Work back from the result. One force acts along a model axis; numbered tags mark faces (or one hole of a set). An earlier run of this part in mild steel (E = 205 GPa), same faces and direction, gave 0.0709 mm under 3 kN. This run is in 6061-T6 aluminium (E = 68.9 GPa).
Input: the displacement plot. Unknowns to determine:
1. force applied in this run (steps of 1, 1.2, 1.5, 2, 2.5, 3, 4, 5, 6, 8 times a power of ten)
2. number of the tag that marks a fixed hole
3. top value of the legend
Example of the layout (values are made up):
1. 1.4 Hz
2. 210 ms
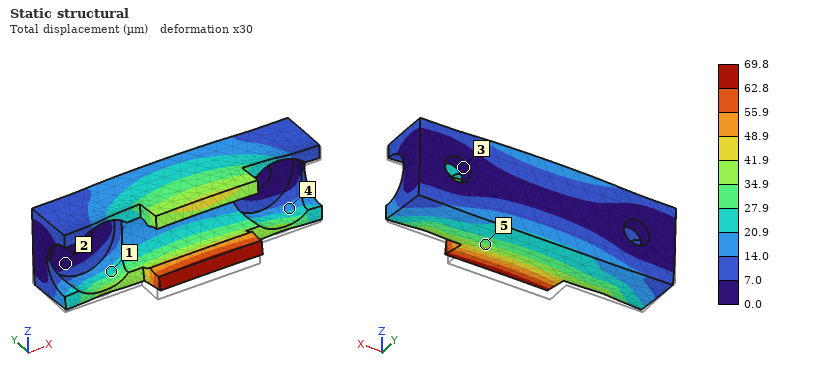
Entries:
1. 1 kN
2. 3
3. 69.8 µm
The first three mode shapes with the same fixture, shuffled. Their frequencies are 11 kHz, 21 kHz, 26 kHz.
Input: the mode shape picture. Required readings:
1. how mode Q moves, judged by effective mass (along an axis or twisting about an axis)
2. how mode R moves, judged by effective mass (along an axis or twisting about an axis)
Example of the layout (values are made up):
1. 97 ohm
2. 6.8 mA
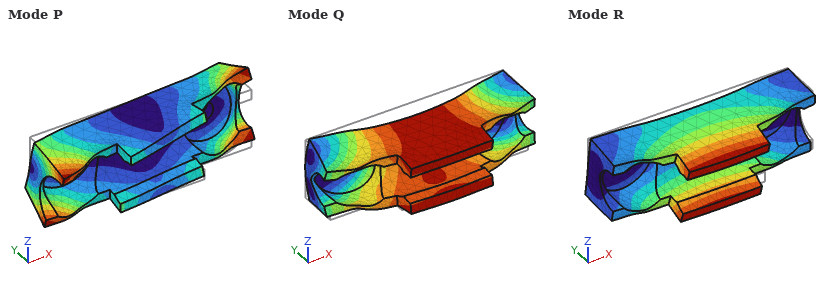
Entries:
1. along Y
2. along Z
